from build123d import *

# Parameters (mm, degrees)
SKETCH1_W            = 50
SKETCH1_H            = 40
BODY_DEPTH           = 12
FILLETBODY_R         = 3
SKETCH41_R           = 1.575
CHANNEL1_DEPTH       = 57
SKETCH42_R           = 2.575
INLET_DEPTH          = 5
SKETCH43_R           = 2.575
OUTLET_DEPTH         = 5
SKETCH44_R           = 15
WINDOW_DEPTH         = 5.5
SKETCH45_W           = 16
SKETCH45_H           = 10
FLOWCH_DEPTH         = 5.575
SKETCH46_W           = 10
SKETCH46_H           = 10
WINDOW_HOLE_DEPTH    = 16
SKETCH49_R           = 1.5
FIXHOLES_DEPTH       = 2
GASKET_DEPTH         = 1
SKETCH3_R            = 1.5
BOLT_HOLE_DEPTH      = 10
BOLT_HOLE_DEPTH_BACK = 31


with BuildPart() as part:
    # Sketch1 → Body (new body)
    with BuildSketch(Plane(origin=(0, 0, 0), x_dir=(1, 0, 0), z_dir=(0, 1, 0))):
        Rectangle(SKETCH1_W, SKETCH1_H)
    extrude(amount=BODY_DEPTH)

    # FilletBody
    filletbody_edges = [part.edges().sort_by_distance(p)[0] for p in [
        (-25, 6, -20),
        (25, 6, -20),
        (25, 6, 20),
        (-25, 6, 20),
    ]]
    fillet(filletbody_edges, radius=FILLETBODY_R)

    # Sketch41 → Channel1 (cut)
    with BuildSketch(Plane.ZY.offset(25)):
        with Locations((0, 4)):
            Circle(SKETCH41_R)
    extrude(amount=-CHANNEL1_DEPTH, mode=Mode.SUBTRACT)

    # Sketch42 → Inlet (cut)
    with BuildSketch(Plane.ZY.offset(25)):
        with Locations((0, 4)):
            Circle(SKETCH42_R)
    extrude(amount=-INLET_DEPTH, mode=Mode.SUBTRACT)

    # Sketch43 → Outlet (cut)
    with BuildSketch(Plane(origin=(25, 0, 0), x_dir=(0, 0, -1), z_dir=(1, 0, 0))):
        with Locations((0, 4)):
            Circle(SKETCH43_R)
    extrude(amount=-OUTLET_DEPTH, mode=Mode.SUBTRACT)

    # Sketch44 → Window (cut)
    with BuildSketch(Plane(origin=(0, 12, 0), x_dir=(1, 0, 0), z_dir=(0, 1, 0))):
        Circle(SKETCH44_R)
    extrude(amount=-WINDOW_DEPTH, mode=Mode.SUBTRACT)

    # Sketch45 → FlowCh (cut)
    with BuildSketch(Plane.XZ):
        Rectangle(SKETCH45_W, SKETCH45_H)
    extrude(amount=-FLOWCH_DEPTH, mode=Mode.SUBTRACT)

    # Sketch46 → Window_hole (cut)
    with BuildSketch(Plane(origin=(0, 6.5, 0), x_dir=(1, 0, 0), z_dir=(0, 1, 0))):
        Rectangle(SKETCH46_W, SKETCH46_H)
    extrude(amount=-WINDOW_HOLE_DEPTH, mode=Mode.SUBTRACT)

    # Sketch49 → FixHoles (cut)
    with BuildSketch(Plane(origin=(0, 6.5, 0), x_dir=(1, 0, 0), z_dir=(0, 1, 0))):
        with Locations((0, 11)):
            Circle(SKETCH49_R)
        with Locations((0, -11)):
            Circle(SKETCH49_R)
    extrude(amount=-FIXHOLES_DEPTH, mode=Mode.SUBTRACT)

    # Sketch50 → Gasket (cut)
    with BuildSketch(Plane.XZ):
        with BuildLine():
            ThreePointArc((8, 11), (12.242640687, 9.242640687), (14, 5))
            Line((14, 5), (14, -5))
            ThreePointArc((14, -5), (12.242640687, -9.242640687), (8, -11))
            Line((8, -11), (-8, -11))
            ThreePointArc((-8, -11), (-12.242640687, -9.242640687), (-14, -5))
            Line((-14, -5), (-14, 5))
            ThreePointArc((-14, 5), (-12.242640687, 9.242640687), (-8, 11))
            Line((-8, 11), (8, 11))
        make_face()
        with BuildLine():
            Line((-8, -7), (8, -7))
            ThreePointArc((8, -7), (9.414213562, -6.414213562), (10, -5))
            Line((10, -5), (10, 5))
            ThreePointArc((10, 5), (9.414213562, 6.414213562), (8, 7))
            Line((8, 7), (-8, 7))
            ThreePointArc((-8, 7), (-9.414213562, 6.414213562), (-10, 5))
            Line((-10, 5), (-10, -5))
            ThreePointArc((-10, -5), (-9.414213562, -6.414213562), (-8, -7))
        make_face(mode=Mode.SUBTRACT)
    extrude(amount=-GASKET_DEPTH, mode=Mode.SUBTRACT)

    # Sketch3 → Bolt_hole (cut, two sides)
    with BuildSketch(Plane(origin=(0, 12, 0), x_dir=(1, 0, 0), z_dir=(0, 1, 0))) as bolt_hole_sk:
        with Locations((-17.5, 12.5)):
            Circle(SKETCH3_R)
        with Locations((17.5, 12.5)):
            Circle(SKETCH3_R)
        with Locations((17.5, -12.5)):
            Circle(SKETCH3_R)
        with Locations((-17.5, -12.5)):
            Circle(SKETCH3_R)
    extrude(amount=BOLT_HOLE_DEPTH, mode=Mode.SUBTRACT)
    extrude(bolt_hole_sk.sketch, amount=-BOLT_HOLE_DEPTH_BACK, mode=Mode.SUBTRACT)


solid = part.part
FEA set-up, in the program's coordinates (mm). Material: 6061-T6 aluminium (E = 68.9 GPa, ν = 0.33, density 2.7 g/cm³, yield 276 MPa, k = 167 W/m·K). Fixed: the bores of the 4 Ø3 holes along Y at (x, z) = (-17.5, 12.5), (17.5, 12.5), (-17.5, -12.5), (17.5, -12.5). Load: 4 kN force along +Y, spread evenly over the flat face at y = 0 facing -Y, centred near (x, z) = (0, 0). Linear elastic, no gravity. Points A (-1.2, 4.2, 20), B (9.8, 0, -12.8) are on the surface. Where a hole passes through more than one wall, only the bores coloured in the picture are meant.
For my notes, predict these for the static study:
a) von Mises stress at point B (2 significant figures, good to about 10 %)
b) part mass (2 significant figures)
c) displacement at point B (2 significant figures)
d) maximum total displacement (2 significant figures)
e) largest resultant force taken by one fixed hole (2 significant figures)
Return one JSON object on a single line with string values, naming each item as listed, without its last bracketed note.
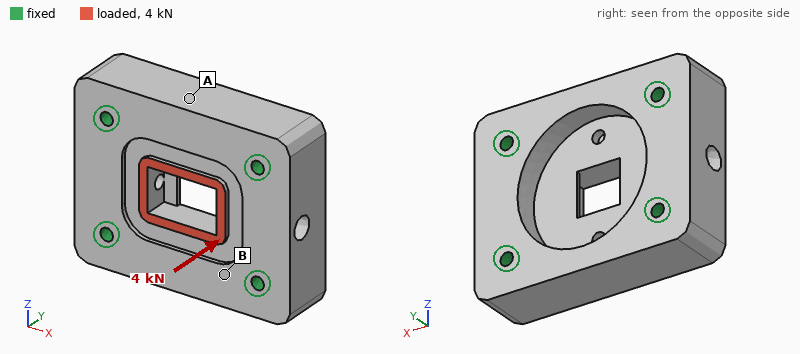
{"von Mises stress at point B": "26 MPa", "part mass": "49 g", "displacement at point B": "4.8 µm", "maximum total displacement": "25 µm", "largest resultant force taken by one fixed hole": "1.0 kN"}
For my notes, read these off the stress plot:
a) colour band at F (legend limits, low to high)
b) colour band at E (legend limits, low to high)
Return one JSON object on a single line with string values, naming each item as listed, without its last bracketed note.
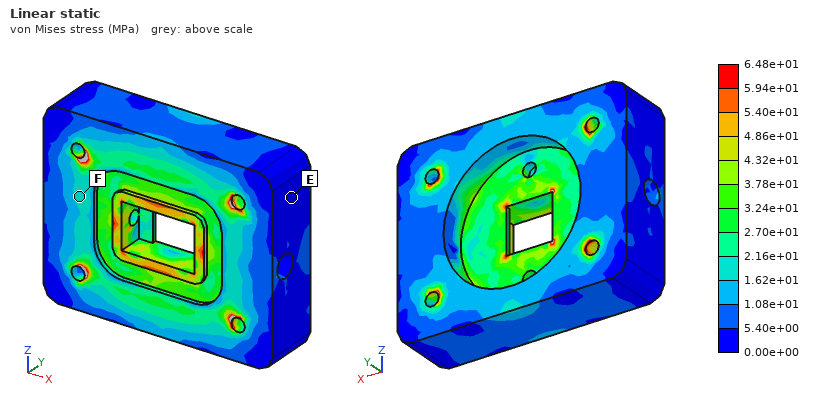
{"colour band at F": "1.62e+01 to 2.16e+01 MPa", "colour band at E": "0.00e+00 to 5.40e+00 MPa"}
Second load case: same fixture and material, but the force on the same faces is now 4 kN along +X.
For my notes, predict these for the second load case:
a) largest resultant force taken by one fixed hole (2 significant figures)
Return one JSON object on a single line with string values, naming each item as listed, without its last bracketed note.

{"largest resultant force taken by one fixed hole": "1.1 kN"}
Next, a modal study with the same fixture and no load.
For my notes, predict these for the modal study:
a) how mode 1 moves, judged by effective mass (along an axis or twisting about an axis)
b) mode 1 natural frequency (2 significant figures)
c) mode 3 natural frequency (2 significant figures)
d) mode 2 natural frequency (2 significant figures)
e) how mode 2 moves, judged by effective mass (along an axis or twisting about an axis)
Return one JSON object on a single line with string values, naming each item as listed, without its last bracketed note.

{"how mode 1 moves, judged by effective mass": "along Y", "mode 1 natural frequency": "30 kHz", "mode 3 natural frequency": "35 kHz", "mode 2 natural frequency": "31 kHz", "how mode 2 moves, judged by effective mass": "twisting about X"}
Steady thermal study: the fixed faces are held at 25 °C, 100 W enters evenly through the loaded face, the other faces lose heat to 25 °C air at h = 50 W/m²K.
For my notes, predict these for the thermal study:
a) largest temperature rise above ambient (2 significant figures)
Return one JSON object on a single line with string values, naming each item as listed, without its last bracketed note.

{"largest temperature rise above ambient": "30 K"}
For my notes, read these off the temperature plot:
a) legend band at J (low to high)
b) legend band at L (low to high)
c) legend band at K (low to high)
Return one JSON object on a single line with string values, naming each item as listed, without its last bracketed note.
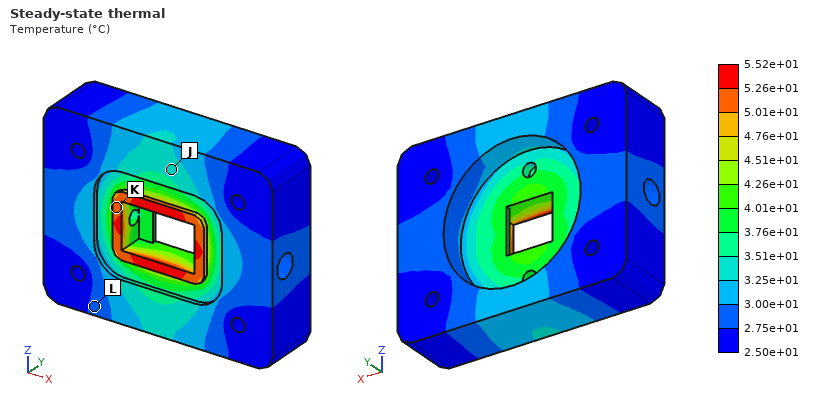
{"legend band at J": "3.25e+01 to 3.51e+01 °C", "legend band at L": "2.75e+01 to 3.00e+01 °C", "legend band at K": "5.01e+01 to 5.26e+01 °C"}
